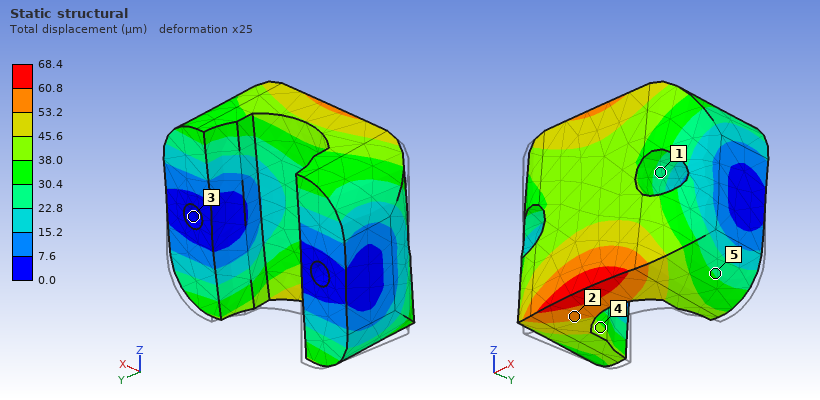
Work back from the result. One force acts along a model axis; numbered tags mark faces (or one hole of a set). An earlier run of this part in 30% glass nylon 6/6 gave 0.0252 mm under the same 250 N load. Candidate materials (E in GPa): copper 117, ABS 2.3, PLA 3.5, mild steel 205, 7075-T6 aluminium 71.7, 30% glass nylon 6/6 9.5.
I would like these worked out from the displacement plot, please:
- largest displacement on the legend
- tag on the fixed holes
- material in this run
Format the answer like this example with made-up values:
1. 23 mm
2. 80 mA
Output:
1. 68.4 µm
2. 3
3. PLA
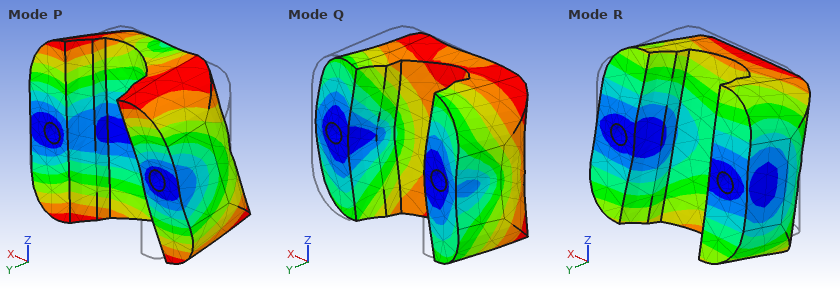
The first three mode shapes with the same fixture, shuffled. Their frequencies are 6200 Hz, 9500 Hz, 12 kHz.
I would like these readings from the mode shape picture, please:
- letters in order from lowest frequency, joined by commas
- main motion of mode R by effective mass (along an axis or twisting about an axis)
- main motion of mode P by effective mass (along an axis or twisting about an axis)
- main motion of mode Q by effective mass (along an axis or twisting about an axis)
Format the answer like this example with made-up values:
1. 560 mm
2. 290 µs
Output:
1. R, P, Q
2. along Z
3. twisting about Y
4. along X
